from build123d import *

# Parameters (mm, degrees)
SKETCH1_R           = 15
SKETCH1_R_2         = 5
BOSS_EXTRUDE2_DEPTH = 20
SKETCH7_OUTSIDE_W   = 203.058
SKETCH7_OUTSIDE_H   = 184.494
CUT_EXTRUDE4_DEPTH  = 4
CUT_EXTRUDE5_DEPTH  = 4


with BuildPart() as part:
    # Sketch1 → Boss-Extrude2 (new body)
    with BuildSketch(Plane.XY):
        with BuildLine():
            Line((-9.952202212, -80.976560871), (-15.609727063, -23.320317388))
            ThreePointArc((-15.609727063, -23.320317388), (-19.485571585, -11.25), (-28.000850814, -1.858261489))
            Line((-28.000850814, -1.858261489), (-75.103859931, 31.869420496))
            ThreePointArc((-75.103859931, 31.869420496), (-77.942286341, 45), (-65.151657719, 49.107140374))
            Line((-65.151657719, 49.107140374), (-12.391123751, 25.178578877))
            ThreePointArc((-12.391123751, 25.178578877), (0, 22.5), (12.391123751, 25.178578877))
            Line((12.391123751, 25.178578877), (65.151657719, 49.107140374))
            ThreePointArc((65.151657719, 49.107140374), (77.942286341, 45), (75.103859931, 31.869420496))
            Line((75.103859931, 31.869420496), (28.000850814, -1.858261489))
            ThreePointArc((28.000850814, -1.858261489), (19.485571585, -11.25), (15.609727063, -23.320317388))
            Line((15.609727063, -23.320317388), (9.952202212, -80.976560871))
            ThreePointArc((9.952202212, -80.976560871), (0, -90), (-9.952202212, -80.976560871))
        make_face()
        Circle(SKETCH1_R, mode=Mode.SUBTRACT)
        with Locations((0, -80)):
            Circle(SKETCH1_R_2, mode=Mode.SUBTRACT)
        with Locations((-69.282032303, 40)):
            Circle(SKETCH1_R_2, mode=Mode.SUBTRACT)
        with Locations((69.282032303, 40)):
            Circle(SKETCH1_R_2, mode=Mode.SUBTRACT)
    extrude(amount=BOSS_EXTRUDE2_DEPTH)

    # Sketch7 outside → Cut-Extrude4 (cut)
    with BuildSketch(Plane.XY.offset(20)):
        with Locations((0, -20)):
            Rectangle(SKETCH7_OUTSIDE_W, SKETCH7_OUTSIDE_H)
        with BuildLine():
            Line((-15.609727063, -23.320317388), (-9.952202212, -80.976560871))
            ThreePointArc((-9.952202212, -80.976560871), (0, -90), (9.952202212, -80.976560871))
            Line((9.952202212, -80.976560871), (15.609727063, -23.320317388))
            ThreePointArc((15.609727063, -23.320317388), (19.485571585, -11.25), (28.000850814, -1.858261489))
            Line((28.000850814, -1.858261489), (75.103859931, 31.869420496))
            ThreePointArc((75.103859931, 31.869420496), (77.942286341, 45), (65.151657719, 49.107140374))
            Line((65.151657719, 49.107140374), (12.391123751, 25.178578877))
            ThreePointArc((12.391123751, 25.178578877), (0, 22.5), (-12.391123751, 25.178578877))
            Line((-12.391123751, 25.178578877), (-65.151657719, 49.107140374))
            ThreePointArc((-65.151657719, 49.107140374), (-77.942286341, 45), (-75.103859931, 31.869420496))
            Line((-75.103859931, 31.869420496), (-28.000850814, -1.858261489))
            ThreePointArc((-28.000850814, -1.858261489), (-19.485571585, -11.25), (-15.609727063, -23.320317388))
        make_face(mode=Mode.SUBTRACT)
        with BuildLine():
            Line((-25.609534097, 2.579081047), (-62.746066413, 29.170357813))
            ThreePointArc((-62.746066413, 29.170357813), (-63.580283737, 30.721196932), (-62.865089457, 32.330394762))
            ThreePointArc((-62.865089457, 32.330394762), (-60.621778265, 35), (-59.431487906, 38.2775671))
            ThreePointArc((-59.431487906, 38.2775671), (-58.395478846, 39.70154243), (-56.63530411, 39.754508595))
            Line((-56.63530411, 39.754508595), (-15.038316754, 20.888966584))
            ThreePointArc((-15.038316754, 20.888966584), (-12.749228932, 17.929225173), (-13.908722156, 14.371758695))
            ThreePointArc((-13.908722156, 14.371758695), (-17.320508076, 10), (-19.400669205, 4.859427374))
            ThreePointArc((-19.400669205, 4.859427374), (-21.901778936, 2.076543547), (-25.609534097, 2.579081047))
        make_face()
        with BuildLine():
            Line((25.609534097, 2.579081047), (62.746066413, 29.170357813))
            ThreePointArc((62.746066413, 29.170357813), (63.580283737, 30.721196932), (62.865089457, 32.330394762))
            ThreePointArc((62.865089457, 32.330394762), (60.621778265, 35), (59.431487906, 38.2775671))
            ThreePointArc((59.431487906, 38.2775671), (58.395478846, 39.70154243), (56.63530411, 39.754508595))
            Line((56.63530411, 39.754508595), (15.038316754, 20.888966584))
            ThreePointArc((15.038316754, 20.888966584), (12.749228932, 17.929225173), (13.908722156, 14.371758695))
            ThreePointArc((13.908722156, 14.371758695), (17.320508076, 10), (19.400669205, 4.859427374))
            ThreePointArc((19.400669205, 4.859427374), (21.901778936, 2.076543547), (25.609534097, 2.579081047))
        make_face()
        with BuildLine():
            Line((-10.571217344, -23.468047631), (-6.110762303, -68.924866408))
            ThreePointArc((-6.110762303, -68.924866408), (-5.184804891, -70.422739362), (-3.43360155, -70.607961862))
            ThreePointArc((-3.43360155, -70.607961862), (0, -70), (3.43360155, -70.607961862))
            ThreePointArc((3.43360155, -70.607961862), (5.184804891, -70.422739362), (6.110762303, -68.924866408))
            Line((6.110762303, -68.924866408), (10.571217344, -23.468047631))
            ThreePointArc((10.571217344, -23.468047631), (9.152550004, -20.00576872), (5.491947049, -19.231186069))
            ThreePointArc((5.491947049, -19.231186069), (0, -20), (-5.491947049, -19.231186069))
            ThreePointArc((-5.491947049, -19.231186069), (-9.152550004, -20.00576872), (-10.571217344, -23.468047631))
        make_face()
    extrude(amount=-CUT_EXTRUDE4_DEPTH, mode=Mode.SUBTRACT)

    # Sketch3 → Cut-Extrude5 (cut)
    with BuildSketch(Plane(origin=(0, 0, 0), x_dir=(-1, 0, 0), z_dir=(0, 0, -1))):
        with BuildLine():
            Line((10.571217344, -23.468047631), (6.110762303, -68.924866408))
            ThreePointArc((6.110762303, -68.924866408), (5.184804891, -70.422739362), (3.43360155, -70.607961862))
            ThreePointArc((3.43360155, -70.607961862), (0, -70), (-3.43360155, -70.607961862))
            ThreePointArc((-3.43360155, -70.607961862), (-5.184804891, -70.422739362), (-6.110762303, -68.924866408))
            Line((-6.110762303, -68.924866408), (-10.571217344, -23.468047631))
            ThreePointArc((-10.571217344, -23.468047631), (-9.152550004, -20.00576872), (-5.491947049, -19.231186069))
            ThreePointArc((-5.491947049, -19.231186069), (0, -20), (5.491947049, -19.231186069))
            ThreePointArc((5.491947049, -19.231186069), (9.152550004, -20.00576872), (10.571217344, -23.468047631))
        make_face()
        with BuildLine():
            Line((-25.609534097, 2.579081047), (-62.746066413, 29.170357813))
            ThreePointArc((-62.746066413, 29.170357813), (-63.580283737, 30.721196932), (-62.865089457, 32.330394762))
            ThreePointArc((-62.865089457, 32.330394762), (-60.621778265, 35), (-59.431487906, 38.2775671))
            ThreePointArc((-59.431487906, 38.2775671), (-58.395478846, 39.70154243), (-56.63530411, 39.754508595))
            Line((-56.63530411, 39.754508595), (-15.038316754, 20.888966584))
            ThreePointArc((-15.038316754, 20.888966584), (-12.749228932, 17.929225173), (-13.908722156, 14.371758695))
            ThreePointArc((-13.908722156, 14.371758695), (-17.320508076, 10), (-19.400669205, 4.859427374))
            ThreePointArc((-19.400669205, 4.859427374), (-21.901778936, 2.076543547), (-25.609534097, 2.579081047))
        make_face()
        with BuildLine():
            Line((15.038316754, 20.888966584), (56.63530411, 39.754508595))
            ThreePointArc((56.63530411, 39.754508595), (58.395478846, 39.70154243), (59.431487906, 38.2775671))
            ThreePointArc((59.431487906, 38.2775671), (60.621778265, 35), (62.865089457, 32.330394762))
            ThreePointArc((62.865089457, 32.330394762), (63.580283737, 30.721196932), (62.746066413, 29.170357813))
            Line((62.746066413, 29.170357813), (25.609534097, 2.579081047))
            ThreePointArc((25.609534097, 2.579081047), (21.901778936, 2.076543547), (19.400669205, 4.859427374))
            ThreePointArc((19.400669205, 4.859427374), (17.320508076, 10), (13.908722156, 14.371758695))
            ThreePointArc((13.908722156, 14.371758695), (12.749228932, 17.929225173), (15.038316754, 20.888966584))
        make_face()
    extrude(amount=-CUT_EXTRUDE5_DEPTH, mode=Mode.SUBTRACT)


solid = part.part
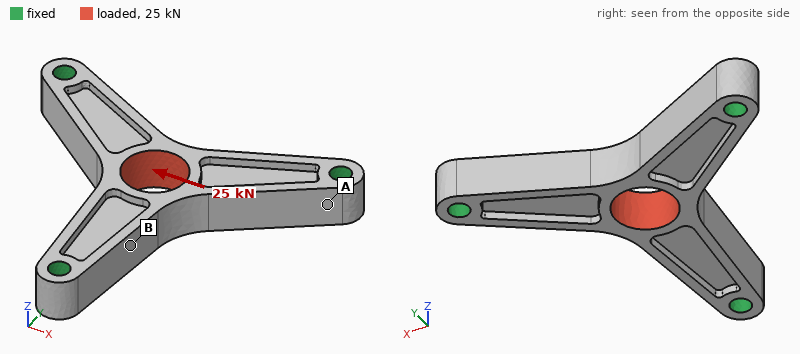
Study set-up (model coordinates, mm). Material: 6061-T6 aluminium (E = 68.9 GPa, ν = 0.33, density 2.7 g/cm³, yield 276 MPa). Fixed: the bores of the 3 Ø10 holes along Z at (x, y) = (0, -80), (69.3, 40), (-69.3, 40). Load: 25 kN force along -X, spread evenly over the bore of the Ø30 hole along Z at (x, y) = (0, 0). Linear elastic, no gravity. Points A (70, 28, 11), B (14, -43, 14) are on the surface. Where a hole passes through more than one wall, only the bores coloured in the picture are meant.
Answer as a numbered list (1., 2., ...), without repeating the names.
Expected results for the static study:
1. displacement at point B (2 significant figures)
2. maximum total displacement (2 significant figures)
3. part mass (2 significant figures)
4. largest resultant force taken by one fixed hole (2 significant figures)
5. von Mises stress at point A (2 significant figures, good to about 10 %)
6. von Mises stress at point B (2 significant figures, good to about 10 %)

1. 42 µm
2. 88 µm
3. 260 g
4. 14 kN
5. 41 MPa
6. 17 MPa
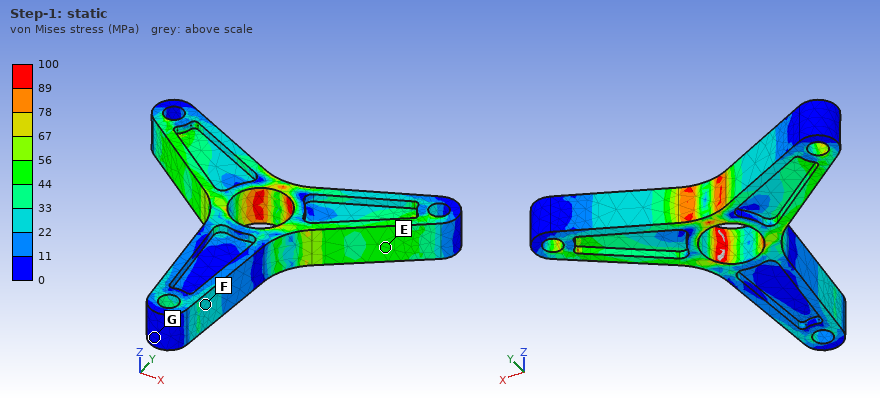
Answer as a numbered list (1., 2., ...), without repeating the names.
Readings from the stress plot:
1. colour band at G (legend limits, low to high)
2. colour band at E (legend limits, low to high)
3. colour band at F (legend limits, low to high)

1. 0 to 11 MPa
2. 44 to 56 MPa
3. 22 to 33 MPa
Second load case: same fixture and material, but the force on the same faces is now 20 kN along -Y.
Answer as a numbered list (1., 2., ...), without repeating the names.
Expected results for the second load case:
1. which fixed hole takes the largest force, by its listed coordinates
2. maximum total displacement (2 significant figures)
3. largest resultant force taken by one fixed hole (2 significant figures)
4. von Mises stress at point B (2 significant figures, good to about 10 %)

1. (0, -80)
2. 75 µm
3. 13 kN
4. 33 MPa
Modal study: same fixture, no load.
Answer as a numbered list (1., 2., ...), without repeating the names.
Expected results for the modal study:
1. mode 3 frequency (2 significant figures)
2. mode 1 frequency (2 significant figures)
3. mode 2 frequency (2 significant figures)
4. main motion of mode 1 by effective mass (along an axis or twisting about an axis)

1. 7500 Hz
2. 3800 Hz
3. 7500 Hz
4. along Z
